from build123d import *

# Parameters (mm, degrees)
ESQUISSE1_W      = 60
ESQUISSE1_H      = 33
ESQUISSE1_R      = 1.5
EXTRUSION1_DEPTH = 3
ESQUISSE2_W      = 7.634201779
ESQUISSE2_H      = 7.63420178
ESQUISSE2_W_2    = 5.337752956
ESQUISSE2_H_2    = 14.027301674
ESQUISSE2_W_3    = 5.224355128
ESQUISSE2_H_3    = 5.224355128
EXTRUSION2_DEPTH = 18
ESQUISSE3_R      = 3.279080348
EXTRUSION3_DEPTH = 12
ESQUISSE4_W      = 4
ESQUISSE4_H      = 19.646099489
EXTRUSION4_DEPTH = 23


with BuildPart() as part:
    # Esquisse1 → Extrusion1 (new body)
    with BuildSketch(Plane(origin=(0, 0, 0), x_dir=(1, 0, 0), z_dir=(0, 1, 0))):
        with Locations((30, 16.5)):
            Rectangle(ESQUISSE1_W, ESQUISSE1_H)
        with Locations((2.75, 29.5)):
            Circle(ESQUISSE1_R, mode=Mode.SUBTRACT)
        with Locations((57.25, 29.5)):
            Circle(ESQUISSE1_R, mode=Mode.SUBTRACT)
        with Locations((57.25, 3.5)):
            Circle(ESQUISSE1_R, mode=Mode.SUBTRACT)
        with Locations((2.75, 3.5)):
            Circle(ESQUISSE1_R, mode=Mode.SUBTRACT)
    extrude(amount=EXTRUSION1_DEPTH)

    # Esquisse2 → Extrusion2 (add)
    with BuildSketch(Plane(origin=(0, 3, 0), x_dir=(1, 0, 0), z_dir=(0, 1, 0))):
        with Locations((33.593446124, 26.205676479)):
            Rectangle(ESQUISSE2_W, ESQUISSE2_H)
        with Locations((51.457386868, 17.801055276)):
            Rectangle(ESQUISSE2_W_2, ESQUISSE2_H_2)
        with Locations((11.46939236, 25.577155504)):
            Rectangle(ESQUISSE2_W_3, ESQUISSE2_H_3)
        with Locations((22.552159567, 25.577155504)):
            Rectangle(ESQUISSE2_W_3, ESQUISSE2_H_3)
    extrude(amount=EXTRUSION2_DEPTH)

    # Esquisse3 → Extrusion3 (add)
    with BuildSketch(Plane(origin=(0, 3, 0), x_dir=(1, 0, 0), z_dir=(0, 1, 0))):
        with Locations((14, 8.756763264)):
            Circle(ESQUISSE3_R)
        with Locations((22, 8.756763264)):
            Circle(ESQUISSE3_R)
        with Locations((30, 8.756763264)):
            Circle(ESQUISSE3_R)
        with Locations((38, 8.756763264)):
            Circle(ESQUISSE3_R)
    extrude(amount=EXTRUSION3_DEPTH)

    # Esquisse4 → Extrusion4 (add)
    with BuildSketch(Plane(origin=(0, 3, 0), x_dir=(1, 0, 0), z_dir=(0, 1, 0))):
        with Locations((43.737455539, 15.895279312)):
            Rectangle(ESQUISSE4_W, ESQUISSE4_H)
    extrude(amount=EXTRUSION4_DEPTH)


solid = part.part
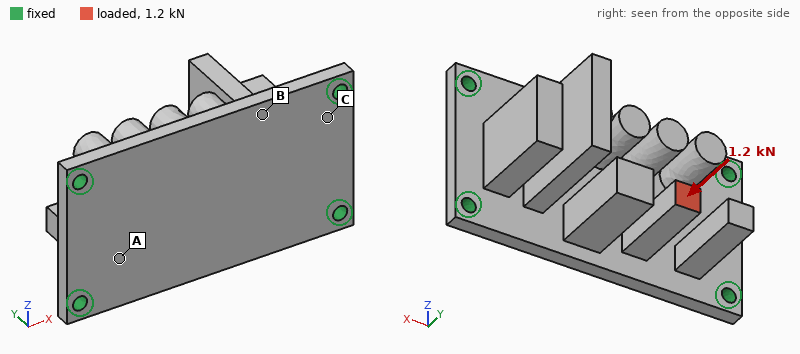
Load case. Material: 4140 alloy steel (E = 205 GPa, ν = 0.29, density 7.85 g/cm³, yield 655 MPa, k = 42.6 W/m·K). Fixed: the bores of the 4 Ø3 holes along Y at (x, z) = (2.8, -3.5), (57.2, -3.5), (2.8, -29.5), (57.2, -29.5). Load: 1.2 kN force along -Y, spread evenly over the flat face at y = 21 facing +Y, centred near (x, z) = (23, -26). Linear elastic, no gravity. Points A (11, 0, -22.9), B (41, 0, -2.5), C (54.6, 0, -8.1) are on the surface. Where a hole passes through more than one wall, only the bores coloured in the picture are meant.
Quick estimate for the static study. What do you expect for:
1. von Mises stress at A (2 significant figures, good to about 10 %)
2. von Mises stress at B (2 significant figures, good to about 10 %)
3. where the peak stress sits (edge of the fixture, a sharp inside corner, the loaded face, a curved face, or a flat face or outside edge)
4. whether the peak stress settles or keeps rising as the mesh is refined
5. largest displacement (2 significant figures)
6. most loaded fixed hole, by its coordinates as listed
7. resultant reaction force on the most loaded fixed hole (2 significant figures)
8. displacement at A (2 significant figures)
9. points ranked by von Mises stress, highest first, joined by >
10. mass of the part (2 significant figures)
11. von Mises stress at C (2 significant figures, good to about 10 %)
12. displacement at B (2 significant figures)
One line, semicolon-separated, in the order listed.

84 MPa; 26 MPa; edge of the fixture; keeps rising; 0.10 mm; (2.8, -29.5); 680 N; 0.028 mm; A > C > B; 99 g; 66 MPa; 0.021 mm
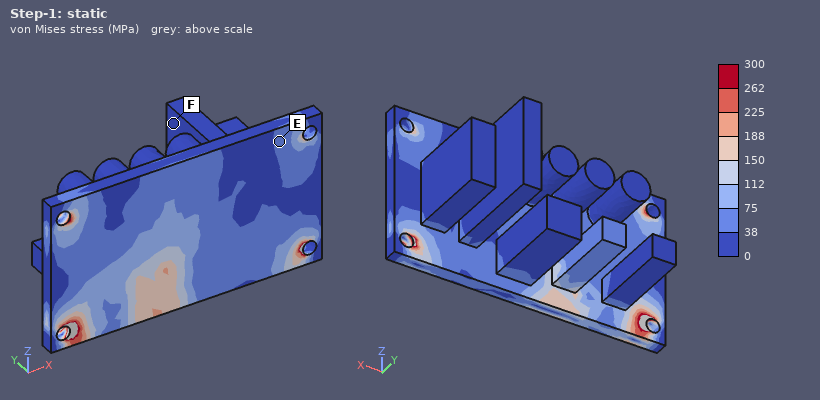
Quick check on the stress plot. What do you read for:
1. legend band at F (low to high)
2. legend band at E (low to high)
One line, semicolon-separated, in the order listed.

0 to 38 MPa; 38 to 75 MPa
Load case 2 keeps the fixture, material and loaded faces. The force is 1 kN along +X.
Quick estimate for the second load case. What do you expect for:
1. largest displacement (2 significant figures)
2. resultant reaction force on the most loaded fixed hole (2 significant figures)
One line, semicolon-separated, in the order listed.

0.32 mm; 570 N
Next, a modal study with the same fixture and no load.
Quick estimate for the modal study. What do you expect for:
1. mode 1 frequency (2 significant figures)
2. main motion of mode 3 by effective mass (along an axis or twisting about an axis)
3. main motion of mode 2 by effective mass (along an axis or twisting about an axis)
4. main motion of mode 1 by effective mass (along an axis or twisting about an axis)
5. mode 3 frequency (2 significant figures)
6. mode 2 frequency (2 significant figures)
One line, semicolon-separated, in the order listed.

2800 Hz; along Y; along Z; along Y; 5200 Hz; 4200 Hz
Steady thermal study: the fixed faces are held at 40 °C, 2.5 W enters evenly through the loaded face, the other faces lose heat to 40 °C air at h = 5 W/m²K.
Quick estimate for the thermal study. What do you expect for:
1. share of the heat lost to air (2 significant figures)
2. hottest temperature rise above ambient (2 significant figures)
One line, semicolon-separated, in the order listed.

8.6 %; 50 K
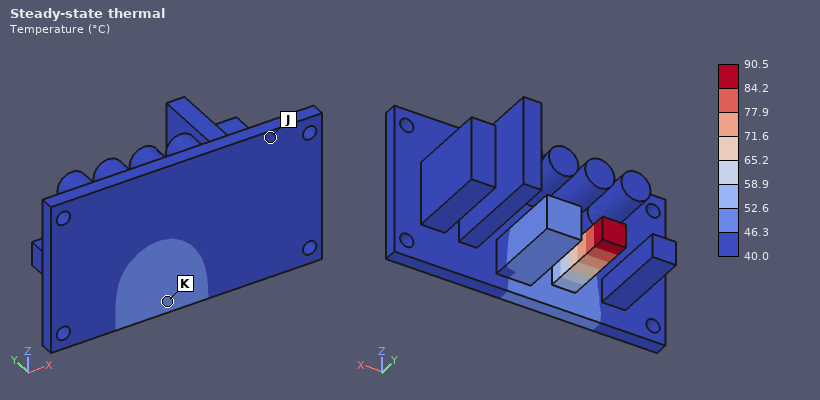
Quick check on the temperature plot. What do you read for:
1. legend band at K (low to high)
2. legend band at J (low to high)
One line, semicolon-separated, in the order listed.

46.3 to 52.6 °C; 40.0 to 46.3 °C
